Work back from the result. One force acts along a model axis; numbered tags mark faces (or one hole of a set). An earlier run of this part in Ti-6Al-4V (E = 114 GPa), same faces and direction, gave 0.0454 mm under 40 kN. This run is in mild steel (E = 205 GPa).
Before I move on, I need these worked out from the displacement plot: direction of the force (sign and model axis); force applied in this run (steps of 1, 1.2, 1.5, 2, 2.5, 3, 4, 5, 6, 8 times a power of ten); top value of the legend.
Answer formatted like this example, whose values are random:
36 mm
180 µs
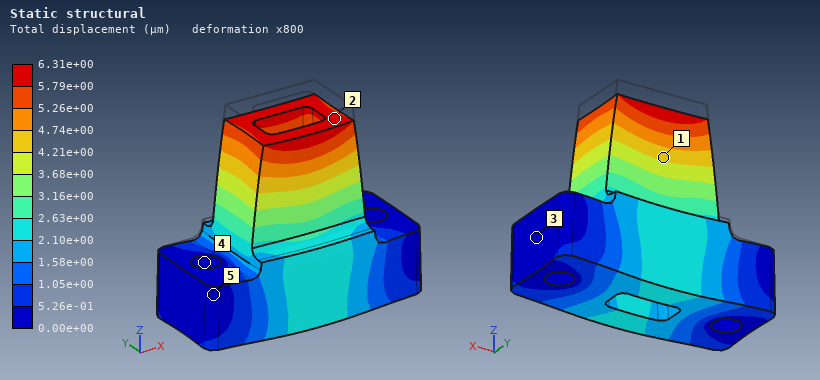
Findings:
-Z
10 kN
6.31e+00 µm
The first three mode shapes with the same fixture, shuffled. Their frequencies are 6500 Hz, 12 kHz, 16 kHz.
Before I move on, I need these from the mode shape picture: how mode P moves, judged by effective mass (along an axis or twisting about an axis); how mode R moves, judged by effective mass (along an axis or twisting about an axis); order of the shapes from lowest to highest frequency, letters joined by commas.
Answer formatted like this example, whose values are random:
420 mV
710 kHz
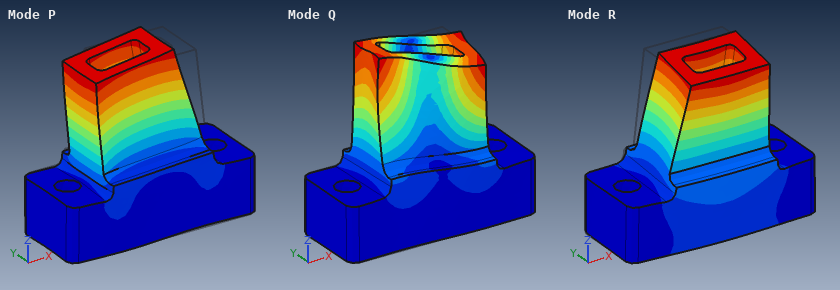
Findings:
along X
along Y
R, P, Q
